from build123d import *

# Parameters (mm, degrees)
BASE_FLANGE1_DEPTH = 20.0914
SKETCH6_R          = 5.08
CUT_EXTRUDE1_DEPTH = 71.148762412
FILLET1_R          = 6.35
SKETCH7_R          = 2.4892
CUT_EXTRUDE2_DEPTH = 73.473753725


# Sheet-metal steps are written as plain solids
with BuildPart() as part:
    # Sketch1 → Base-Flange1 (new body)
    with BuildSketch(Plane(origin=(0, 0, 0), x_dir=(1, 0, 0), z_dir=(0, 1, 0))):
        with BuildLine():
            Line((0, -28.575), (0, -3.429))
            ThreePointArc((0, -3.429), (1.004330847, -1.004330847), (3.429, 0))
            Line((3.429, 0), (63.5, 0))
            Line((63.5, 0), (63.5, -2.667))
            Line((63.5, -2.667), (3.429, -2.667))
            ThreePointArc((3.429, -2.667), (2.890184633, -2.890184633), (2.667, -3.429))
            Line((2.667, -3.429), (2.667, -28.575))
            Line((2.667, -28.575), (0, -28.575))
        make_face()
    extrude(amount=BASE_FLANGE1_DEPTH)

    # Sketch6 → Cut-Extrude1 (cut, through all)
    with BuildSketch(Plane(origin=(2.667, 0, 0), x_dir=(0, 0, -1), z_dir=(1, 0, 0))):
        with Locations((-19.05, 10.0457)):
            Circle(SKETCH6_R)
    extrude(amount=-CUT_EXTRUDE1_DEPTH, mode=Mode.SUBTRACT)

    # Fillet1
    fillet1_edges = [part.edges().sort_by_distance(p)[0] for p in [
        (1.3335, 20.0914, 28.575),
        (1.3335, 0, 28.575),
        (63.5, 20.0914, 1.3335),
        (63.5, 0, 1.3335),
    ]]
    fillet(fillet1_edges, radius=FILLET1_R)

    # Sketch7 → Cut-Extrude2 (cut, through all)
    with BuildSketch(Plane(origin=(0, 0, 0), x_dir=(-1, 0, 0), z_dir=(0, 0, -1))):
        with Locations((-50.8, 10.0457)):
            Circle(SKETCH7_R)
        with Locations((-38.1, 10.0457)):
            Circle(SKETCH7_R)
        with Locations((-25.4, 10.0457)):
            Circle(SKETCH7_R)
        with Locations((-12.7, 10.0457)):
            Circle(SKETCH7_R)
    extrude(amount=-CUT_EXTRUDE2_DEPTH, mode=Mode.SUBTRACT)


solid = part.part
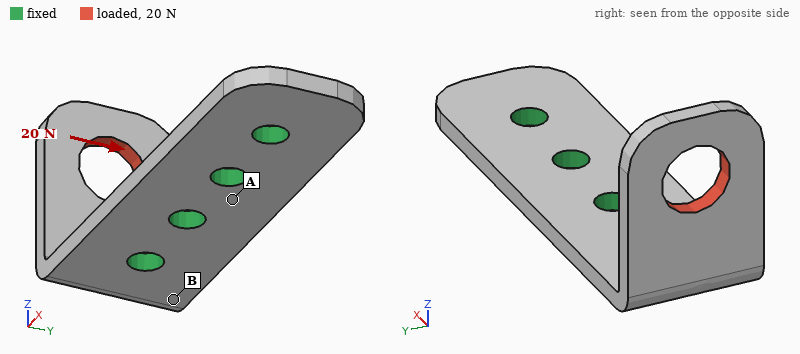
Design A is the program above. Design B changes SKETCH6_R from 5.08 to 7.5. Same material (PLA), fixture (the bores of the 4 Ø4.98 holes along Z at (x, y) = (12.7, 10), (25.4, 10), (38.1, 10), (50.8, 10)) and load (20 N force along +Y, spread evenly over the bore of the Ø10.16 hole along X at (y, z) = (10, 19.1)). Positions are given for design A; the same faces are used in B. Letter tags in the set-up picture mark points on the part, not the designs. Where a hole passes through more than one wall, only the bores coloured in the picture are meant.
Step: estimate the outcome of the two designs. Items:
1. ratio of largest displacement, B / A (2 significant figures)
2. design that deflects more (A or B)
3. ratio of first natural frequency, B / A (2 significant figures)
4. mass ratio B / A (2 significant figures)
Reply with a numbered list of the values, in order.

1. 1.1
2. B
3. 1.2
4. 0.94
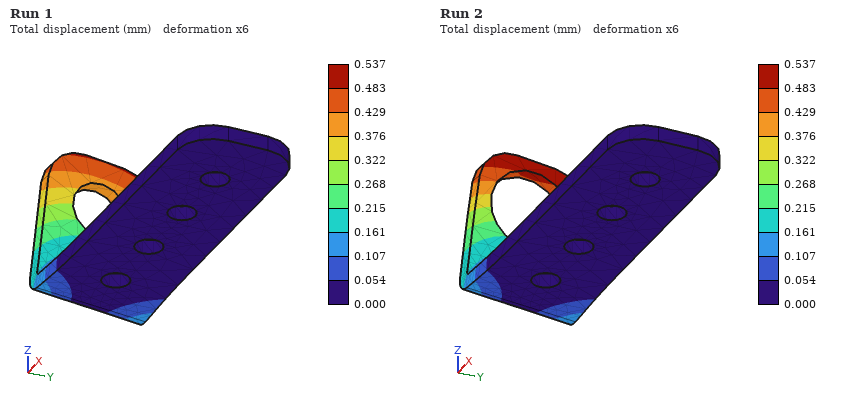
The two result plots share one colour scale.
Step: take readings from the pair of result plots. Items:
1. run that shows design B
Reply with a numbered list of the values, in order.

1. Run 2
